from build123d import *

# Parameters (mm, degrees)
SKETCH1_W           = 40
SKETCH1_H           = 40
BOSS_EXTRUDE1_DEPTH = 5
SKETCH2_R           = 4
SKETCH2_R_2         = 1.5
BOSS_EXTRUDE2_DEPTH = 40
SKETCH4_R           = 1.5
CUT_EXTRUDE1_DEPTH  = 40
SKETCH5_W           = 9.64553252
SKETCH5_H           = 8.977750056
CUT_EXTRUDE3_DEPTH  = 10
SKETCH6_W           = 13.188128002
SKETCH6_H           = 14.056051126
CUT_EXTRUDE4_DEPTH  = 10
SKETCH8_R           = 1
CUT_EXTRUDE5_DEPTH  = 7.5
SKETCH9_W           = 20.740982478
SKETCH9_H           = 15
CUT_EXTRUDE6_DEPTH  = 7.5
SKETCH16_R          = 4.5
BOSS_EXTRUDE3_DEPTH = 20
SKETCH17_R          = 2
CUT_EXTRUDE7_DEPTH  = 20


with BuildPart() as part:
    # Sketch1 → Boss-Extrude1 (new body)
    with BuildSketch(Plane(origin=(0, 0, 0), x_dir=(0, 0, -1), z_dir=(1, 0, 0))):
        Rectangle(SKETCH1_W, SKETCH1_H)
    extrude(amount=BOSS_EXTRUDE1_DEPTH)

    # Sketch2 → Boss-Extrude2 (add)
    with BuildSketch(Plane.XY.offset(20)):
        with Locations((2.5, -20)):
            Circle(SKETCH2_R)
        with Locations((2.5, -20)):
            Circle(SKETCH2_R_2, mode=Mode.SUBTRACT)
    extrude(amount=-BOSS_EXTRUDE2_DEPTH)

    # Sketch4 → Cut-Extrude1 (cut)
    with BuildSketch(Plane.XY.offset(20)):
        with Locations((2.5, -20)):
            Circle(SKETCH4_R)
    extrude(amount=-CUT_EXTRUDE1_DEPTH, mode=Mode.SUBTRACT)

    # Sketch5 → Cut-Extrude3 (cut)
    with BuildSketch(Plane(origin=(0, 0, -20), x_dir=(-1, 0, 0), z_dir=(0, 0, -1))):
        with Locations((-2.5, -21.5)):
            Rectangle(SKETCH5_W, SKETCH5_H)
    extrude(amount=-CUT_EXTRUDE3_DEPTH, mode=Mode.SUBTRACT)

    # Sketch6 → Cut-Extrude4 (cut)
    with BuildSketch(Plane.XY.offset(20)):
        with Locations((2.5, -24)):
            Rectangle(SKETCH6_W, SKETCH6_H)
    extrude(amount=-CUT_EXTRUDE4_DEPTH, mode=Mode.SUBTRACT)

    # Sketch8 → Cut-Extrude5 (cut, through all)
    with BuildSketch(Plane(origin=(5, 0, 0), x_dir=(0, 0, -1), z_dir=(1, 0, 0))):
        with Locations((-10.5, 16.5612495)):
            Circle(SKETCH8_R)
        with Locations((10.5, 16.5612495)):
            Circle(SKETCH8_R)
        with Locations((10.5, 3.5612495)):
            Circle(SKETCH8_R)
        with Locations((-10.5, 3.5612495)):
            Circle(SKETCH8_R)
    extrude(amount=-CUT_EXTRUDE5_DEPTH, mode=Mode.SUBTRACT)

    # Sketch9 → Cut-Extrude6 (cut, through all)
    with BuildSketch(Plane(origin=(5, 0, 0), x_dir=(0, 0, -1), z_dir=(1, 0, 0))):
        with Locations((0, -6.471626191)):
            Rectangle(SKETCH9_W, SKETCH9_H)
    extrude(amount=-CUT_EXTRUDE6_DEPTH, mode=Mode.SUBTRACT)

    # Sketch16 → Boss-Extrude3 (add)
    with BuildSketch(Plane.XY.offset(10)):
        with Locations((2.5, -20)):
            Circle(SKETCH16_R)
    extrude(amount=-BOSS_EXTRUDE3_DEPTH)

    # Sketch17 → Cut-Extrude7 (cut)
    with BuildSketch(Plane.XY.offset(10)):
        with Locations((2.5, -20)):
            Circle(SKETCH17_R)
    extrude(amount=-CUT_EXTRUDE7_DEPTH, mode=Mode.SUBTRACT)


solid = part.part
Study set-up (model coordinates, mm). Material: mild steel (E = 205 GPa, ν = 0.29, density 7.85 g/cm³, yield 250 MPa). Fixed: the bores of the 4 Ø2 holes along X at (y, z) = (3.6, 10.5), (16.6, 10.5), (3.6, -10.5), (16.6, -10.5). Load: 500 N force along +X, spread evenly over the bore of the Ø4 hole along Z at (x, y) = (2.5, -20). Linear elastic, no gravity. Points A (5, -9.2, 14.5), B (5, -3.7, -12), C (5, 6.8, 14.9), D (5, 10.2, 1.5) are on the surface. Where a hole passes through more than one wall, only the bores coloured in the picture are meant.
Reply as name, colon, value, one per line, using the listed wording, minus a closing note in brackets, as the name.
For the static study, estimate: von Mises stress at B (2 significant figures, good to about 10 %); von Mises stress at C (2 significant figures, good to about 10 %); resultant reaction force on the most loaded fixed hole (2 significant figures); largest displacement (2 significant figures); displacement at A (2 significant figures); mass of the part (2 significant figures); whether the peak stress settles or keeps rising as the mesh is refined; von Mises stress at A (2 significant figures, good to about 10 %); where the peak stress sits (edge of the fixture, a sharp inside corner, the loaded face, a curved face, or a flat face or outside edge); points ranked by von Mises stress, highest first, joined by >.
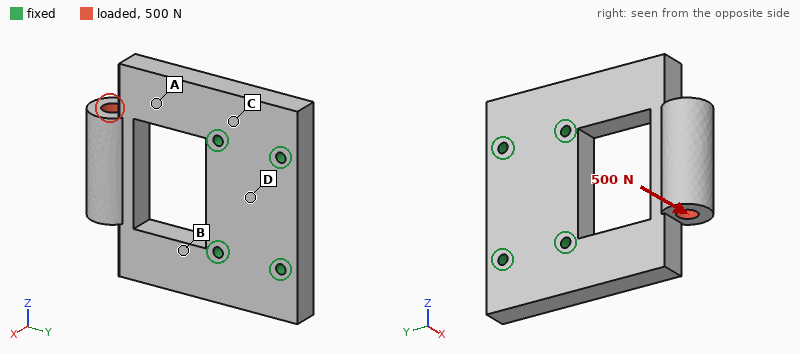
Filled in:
von Mises stress at B: 110 MPa
von Mises stress at C: 46 MPa
resultant reaction force on the most loaded fixed hole: 450 N
largest displacement: 99 µm
displacement at A: 26 µm
mass of the part: 52 g
whether the peak stress settles or keeps rising as the mesh is refined: keeps rising
von Mises stress at A: 76 MPa
where the peak stress sits: edge of the fixture
points ranked by von Mises stress, highest first, joined by >: B > A > C > D
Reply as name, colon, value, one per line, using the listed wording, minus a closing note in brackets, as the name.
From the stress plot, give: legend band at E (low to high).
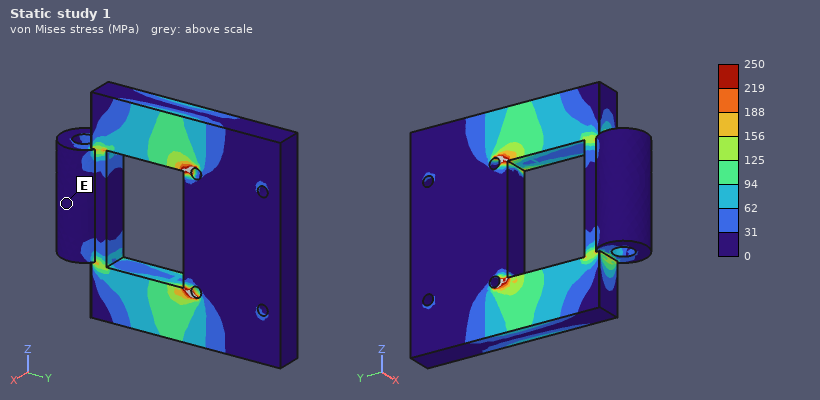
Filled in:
legend band at E: 0 to 31 MPa
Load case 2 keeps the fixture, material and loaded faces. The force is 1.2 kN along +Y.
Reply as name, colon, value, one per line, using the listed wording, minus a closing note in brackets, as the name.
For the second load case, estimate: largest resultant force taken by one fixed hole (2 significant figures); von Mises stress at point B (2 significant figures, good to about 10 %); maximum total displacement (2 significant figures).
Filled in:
largest resultant force taken by one fixed hole: 520 N
von Mises stress at point B: 22 MPa
maximum total displacement: 7.1 µm
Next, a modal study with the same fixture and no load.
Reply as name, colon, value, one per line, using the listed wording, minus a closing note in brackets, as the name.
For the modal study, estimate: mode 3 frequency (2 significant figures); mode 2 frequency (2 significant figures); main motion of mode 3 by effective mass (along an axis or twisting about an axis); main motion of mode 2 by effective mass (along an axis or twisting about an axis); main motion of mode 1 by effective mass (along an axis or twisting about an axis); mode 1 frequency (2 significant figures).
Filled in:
mode 3 frequency: 9500 Hz
mode 2 frequency: 8900 Hz
main motion of mode 3 by effective mass: along Z
main motion of mode 2 by effective mass: twisting about Y
main motion of mode 1 by effective mass: along X
mode 1 frequency: 3900 Hz
